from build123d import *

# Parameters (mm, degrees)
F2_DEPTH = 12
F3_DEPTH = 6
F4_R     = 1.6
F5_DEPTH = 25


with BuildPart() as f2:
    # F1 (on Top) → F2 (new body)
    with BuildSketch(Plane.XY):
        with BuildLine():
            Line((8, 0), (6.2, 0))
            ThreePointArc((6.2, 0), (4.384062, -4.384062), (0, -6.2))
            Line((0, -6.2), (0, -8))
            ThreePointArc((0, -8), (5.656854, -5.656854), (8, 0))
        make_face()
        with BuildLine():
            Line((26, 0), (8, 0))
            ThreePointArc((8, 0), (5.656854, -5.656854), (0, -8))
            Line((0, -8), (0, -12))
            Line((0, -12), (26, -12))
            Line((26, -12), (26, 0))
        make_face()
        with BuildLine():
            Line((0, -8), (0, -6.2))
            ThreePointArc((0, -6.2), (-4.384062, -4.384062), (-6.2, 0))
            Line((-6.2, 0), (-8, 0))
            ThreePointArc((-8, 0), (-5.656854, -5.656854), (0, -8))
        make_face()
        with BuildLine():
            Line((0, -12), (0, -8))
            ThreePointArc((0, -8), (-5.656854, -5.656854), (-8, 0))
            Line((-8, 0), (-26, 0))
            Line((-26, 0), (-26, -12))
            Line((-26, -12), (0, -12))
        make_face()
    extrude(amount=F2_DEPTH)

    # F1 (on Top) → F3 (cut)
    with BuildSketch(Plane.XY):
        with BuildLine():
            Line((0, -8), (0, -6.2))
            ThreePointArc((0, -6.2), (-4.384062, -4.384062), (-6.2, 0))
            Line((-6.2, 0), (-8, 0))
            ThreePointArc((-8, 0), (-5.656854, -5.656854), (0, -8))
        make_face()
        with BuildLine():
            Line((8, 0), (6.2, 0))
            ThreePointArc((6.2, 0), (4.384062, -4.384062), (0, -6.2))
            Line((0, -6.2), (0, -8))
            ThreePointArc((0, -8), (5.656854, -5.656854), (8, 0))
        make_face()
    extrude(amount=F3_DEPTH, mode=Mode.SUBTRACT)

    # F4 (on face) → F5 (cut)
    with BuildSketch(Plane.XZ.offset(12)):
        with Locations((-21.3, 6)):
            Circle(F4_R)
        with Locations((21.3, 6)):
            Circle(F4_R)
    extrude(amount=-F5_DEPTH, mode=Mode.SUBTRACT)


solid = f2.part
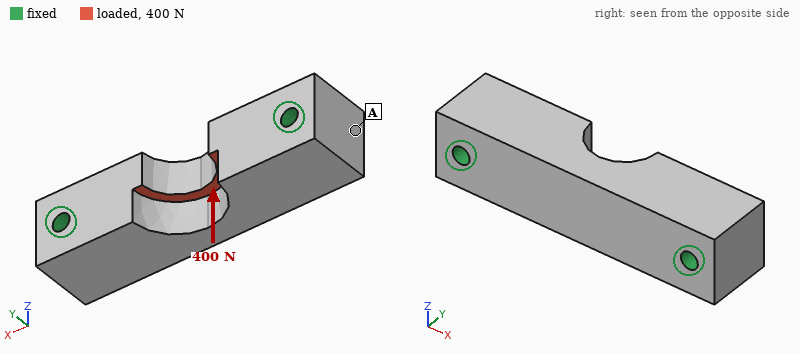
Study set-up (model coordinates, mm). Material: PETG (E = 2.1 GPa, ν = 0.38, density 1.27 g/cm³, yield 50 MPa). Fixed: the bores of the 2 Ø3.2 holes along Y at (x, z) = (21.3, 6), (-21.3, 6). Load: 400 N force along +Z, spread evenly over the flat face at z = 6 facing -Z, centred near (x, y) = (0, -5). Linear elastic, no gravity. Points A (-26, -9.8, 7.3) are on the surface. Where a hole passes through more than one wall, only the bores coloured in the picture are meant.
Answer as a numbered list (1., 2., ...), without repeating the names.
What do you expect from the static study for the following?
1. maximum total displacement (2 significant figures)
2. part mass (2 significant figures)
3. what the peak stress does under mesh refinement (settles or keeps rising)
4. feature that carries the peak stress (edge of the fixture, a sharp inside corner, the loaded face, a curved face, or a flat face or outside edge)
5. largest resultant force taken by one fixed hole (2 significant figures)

1. 0.17 mm
2. 8.0 g
3. keeps rising
4. edge of the fixture
5. 200 N
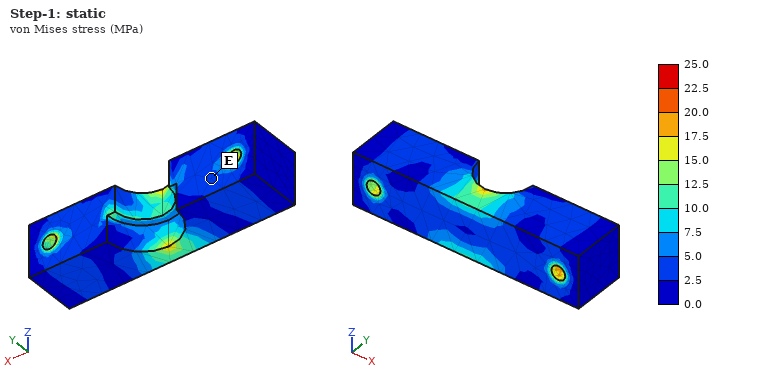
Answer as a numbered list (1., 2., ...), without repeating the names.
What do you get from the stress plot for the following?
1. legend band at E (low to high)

1. 2.5 to 5.0 MPa
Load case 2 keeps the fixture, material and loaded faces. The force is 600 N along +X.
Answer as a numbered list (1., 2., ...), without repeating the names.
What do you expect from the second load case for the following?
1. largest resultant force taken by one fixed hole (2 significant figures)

1. 300 N
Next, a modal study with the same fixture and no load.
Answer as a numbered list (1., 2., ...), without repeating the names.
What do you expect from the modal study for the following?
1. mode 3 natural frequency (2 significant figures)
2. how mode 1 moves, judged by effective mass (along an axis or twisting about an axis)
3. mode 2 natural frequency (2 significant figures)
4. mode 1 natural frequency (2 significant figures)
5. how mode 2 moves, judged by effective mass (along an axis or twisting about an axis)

1. 10000 Hz
2. along Z
3. 6300 Hz
4. 4900 Hz
5. along Y
